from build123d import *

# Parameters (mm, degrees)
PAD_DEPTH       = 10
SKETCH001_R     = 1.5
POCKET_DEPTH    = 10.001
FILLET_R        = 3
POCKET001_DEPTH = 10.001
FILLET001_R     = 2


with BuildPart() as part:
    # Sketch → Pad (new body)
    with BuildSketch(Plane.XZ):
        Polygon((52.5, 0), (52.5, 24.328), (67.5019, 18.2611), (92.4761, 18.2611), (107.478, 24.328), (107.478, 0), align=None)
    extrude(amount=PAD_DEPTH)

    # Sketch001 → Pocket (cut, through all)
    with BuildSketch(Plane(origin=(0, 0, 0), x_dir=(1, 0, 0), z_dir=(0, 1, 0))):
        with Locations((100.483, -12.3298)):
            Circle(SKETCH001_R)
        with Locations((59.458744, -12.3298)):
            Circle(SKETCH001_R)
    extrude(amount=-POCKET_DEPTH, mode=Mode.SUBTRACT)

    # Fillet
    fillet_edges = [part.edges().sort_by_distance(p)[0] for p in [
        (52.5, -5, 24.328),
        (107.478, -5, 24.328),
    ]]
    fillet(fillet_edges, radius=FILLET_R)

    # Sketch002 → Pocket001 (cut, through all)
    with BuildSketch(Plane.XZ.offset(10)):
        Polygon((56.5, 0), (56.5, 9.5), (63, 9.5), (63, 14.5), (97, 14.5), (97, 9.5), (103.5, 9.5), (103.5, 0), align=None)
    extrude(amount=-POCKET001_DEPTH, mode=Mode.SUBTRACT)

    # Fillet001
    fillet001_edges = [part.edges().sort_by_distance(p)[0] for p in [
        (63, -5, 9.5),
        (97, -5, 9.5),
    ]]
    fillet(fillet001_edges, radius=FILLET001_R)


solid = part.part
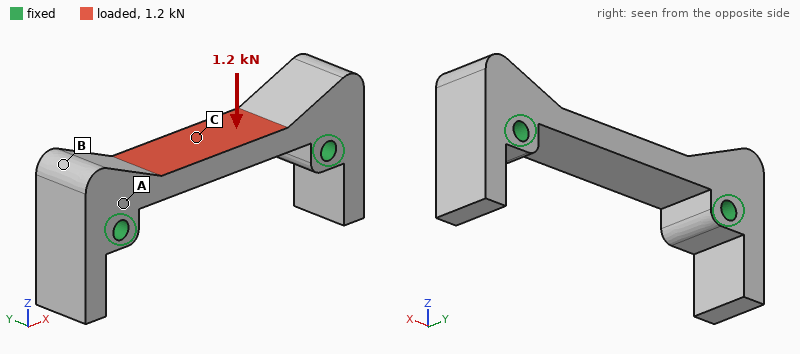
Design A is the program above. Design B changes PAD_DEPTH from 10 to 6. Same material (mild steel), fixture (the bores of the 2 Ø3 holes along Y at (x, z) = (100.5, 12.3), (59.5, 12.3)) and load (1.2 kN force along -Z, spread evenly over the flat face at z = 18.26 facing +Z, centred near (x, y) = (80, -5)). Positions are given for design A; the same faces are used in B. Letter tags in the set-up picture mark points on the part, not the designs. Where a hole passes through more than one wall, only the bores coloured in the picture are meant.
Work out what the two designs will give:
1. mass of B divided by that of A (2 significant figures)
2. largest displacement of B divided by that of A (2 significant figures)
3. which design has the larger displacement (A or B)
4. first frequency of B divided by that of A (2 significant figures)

0.60
1.7
B
0.99
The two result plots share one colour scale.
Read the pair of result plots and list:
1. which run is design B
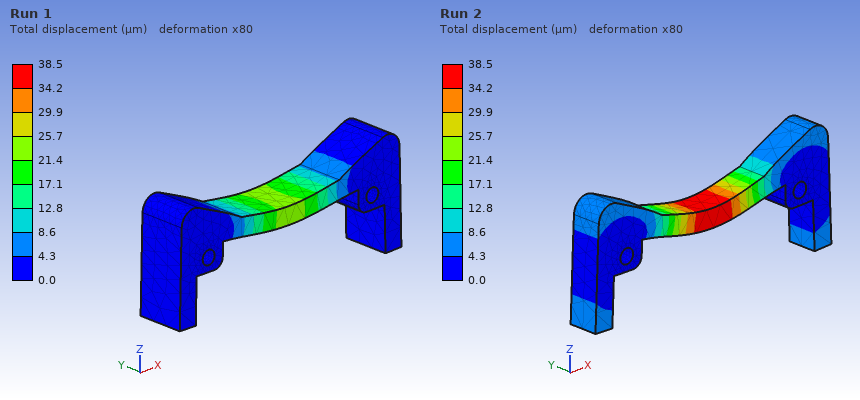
Run 2
